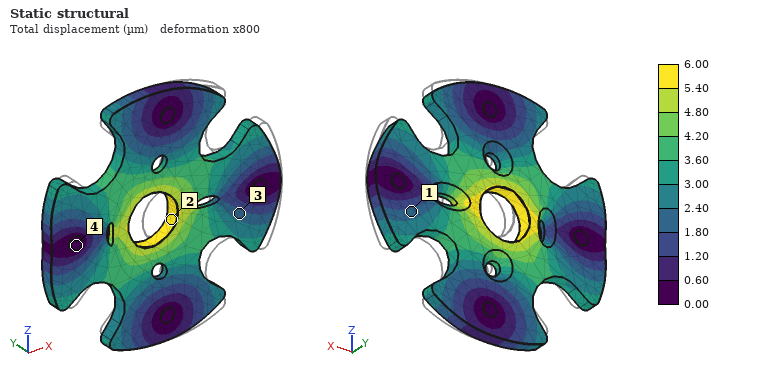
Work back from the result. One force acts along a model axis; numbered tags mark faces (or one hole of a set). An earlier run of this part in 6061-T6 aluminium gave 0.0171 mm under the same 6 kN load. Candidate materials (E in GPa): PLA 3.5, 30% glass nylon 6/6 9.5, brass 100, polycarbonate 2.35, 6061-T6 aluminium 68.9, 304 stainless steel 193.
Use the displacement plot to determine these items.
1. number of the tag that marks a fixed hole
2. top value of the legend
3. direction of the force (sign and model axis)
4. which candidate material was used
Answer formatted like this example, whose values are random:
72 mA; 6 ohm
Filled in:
4; 6.00 µm; -X; 304 stainless steel
